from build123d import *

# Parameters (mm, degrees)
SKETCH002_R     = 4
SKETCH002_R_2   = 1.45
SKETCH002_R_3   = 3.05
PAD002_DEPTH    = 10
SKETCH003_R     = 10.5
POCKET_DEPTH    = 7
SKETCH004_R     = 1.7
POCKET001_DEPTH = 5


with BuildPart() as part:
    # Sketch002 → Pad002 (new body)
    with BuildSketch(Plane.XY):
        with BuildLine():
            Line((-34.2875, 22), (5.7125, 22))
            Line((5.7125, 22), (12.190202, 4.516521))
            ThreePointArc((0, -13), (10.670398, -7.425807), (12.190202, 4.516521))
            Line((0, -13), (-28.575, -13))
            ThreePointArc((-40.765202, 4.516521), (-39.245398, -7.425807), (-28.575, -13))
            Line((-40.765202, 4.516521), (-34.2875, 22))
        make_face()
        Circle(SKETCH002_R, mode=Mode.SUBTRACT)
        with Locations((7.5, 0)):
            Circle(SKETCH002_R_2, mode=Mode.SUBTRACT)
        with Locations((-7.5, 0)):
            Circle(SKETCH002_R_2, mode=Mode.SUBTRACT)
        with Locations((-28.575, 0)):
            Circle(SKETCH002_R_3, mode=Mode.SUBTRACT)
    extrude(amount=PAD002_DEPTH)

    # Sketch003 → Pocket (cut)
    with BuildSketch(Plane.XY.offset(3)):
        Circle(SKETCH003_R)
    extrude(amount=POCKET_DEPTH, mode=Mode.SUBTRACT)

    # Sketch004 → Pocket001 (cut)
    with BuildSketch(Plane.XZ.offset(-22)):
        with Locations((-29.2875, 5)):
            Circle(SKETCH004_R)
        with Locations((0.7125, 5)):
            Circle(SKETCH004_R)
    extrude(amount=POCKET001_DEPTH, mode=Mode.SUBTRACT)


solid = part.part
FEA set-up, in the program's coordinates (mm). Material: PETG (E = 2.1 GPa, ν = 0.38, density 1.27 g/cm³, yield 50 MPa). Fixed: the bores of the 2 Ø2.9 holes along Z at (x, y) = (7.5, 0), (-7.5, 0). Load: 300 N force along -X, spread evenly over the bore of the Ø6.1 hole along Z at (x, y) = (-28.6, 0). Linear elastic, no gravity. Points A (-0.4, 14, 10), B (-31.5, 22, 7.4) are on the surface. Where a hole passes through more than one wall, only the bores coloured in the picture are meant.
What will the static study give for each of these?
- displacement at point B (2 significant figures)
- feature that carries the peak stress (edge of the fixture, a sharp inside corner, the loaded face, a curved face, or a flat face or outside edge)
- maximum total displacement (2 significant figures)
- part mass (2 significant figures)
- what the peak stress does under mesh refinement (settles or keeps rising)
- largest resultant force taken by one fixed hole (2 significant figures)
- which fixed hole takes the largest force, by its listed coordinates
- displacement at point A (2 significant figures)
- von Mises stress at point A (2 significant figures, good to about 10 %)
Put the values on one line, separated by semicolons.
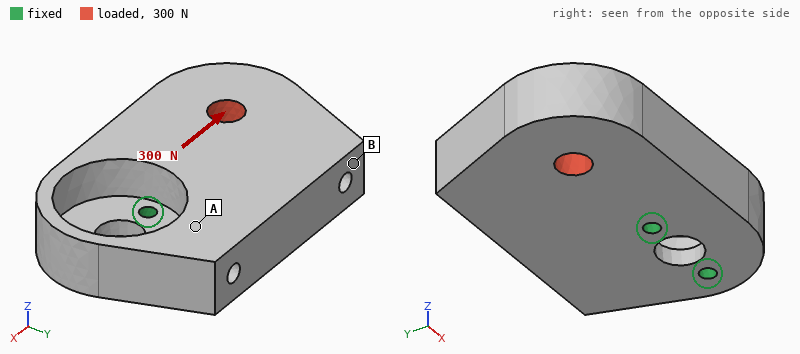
0.16 mm; edge of the fixture; 0.25 mm; 18 g; keeps rising; 220 N; (-7.5, 0); 0.058 mm; 2.2 MPa
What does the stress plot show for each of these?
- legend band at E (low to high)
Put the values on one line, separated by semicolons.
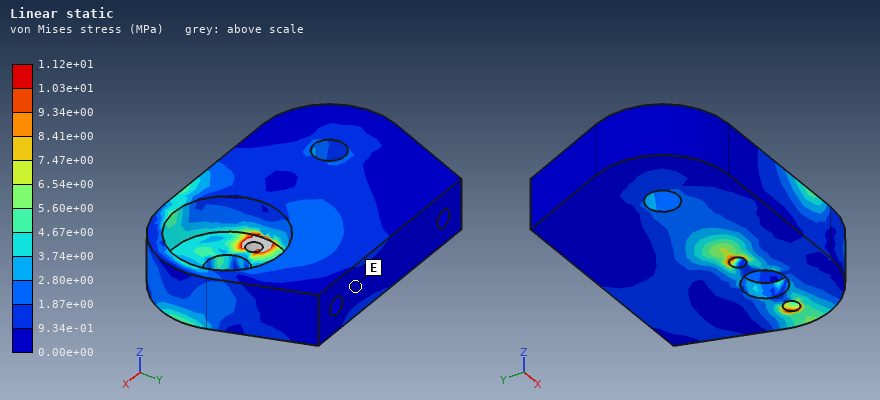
0.00e+00 to 9.34e-01 MPa
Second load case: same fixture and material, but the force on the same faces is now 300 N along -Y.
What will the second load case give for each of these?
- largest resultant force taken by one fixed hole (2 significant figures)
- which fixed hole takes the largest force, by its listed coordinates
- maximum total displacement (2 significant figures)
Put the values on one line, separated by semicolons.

640 N; (-7.5, 0); 0.65 mm
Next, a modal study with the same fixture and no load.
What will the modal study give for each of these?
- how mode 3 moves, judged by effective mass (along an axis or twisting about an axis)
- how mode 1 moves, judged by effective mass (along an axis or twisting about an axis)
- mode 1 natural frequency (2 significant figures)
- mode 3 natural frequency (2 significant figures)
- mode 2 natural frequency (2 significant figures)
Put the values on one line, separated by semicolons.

along Y; along Z; 730 Hz; 1500 Hz; 940 Hz
